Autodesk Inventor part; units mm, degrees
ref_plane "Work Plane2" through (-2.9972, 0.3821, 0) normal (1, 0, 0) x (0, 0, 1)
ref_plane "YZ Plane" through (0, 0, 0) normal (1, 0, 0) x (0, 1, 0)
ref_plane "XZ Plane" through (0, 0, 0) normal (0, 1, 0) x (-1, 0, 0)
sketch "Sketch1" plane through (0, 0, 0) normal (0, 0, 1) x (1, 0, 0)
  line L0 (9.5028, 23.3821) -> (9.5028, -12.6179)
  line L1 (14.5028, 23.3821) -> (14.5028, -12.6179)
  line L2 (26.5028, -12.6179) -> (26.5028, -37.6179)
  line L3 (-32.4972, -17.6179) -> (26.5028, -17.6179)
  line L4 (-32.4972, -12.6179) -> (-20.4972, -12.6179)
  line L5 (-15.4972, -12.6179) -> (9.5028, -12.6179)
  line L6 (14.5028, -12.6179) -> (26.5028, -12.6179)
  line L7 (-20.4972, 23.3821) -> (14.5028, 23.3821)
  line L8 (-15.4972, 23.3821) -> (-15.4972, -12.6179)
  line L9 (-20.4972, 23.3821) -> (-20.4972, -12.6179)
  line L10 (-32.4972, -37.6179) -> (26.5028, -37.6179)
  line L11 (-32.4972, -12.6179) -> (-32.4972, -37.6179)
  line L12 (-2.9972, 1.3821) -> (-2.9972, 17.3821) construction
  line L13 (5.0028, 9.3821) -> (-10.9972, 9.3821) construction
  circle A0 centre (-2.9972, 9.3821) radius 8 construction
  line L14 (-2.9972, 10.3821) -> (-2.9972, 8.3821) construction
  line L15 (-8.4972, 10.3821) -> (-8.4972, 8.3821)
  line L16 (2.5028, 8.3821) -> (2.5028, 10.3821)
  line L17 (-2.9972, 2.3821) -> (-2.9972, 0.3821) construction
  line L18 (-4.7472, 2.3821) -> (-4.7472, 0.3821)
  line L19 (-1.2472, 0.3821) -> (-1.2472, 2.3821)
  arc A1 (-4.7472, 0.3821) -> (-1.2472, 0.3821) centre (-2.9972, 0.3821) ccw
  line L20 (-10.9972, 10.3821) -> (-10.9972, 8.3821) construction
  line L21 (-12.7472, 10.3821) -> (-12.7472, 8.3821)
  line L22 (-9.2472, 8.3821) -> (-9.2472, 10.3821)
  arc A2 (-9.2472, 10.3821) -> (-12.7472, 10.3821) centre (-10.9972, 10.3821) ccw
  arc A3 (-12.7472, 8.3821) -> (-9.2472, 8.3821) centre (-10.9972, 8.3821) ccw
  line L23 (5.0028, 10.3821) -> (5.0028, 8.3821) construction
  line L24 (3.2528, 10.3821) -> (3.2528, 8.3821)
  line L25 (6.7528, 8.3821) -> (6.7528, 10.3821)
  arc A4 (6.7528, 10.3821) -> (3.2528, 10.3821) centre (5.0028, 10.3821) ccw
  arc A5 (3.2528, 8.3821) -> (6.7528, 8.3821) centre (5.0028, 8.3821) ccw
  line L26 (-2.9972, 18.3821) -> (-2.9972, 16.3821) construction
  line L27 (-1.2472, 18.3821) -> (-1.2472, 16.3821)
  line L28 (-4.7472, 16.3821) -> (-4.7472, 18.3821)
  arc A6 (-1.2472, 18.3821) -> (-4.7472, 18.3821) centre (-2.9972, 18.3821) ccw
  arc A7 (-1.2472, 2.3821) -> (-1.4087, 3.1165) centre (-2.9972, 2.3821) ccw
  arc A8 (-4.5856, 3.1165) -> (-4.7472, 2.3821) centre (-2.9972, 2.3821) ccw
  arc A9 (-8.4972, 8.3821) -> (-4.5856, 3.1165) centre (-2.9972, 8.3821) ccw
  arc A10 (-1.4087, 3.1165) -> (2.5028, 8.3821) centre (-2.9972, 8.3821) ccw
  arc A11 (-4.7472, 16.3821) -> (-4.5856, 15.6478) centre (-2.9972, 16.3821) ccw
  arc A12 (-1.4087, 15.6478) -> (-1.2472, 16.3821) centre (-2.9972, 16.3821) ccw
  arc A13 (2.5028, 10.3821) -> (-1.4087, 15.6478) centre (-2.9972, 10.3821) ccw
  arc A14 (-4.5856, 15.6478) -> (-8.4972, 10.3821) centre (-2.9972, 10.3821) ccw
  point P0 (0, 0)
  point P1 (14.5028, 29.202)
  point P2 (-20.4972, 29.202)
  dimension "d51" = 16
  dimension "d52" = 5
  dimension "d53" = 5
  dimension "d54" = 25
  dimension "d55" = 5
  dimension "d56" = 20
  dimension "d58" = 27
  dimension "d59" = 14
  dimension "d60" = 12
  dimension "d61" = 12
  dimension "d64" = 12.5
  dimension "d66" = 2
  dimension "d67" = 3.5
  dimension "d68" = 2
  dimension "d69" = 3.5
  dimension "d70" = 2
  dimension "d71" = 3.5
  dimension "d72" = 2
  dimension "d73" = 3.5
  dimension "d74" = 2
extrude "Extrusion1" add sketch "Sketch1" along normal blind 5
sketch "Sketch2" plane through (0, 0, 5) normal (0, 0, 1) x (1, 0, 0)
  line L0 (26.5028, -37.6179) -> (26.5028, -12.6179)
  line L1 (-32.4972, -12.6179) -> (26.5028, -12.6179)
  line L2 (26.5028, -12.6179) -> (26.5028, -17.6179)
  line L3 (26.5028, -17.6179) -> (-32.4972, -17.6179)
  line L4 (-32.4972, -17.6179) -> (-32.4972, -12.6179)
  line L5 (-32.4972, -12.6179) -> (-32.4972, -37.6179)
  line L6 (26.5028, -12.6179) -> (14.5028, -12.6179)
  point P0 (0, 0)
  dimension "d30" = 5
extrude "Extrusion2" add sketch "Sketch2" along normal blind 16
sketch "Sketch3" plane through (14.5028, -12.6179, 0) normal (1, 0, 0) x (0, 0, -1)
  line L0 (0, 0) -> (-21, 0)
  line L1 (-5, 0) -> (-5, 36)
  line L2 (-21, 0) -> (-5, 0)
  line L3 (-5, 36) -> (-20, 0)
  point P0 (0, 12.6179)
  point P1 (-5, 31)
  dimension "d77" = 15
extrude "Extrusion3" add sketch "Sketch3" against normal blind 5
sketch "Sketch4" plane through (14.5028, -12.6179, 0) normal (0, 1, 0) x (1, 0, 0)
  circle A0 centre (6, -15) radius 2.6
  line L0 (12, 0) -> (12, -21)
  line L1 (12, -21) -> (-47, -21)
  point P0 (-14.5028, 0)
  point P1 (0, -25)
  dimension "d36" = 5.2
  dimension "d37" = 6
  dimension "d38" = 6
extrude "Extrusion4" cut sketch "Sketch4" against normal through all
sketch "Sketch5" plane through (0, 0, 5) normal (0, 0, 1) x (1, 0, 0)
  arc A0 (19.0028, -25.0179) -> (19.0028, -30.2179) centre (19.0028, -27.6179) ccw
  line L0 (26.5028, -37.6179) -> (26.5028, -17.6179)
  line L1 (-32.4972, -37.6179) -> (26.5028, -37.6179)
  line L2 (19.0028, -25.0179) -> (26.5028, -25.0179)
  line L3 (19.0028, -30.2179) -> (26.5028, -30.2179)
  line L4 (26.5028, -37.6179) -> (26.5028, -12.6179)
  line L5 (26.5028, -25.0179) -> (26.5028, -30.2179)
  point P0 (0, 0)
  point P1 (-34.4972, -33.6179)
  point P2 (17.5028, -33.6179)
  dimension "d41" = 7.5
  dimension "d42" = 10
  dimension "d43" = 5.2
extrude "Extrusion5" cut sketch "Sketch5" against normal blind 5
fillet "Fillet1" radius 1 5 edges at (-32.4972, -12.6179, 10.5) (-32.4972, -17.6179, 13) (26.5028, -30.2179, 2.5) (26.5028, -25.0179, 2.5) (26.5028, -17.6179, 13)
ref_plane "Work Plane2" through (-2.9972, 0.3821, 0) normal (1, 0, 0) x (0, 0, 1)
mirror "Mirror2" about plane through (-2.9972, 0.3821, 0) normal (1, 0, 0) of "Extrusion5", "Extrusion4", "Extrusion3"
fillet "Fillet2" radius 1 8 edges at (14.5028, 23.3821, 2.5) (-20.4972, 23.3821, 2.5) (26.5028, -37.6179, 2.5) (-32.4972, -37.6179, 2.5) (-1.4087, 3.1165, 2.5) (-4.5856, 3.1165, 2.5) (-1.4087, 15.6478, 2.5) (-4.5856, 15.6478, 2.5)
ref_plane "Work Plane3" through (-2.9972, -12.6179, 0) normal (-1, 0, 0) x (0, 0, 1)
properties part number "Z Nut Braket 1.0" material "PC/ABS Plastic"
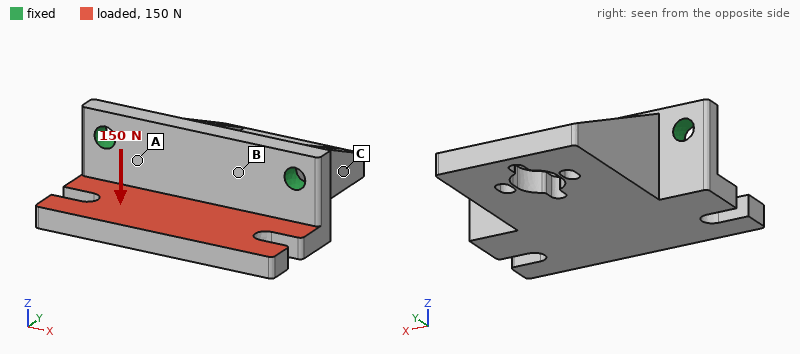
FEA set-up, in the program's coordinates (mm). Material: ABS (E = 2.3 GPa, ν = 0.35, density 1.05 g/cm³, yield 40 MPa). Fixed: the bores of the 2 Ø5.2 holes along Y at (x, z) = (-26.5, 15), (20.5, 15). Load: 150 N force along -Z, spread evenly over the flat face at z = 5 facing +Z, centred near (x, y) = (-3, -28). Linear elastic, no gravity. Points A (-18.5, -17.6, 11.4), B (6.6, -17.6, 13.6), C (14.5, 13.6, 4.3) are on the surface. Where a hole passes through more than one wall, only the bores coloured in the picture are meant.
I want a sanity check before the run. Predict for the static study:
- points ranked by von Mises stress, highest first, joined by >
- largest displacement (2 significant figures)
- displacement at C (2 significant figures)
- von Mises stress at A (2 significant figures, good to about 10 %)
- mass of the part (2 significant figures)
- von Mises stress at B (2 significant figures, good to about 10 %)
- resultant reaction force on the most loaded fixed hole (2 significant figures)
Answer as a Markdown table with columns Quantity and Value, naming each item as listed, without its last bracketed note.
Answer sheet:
| Quantity | Value |
|---|---|
| points ranked by von Mises stress, highest first, joined by > | A > B > C |
| largest displacement | 0.52 mm |
| displacement at C | 0.26 mm |
| von Mises stress at A | 4.8 MPa |
| mass of the part | 20 g |
| von Mises stress at B | 2.3 MPa |
| resultant reaction force on the most loaded fixed hole | 87 N |
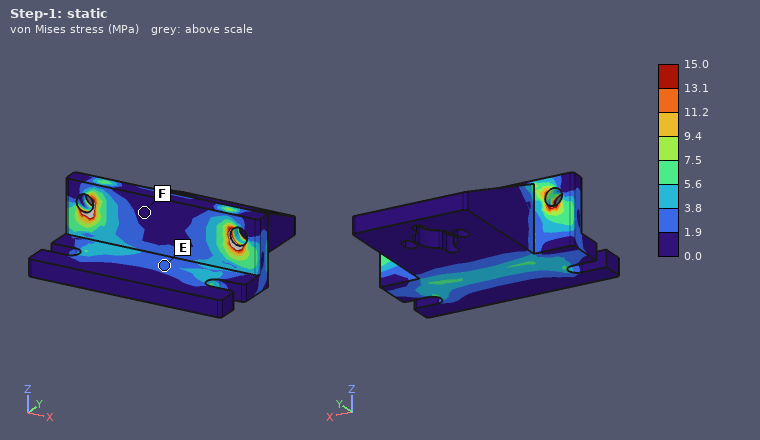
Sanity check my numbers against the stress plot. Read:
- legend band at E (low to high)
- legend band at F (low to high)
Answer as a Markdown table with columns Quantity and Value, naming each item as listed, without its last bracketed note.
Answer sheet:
| Quantity | Value |
|---|---|
| legend band at E | 1.9 to 3.8 MPa |
| legend band at F | 0.0 to 1.9 MPa |
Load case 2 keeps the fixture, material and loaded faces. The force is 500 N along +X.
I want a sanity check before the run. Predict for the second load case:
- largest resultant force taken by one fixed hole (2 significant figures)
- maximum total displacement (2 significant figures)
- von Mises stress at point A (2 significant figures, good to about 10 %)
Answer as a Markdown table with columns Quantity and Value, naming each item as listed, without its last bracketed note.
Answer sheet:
| Quantity | Value |
|---|---|
| largest resultant force taken by one fixed hole | 300 N |
| maximum total displacement | 0.40 mm |
| von Mises stress at point A | 6.7 MPa |
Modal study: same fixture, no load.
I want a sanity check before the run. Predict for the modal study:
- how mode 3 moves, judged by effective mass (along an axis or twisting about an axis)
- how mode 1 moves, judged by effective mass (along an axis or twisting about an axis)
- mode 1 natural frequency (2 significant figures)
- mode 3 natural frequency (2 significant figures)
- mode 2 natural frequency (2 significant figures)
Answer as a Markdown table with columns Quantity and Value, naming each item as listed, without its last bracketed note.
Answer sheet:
| Quantity | Value |
|---|---|
| how mode 3 moves, judged by effective mass | along Z |
| how mode 1 moves, judged by effective mass | along Y |
| mode 1 natural frequency | 880 Hz |
| mode 3 natural frequency | 2100 Hz |
| mode 2 natural frequency | 1700 Hz |
